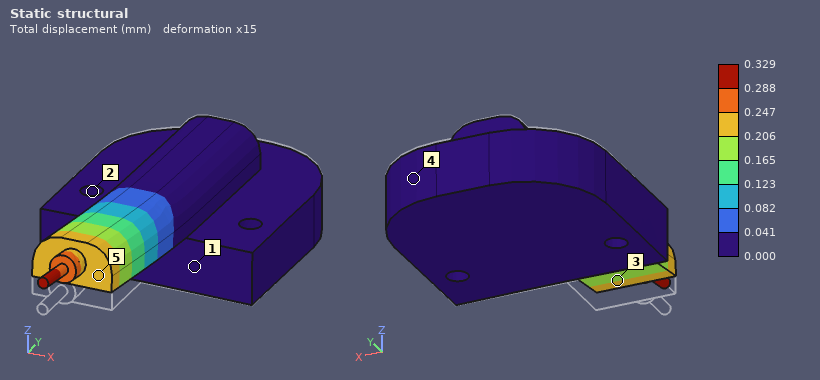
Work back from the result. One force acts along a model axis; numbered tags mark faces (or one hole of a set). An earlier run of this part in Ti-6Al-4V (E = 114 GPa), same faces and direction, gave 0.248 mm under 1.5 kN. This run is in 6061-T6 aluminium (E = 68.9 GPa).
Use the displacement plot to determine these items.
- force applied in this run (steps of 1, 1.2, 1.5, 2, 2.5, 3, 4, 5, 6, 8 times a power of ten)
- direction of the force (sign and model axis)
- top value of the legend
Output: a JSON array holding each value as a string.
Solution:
["1.2 kN", "+Z", "0.329 mm"]
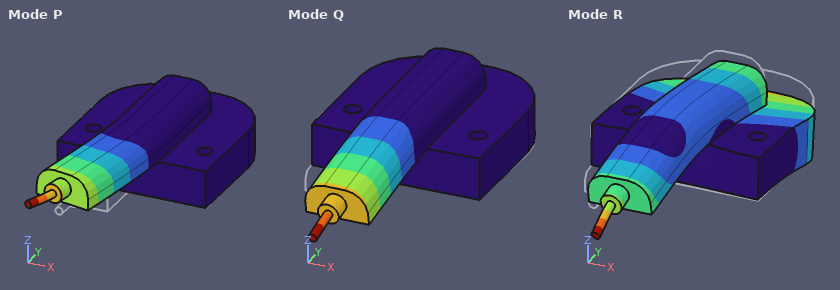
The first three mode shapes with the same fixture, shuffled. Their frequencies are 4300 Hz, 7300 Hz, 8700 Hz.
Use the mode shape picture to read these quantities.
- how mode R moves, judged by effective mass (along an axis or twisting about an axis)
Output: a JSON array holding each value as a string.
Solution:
["along Z"]
